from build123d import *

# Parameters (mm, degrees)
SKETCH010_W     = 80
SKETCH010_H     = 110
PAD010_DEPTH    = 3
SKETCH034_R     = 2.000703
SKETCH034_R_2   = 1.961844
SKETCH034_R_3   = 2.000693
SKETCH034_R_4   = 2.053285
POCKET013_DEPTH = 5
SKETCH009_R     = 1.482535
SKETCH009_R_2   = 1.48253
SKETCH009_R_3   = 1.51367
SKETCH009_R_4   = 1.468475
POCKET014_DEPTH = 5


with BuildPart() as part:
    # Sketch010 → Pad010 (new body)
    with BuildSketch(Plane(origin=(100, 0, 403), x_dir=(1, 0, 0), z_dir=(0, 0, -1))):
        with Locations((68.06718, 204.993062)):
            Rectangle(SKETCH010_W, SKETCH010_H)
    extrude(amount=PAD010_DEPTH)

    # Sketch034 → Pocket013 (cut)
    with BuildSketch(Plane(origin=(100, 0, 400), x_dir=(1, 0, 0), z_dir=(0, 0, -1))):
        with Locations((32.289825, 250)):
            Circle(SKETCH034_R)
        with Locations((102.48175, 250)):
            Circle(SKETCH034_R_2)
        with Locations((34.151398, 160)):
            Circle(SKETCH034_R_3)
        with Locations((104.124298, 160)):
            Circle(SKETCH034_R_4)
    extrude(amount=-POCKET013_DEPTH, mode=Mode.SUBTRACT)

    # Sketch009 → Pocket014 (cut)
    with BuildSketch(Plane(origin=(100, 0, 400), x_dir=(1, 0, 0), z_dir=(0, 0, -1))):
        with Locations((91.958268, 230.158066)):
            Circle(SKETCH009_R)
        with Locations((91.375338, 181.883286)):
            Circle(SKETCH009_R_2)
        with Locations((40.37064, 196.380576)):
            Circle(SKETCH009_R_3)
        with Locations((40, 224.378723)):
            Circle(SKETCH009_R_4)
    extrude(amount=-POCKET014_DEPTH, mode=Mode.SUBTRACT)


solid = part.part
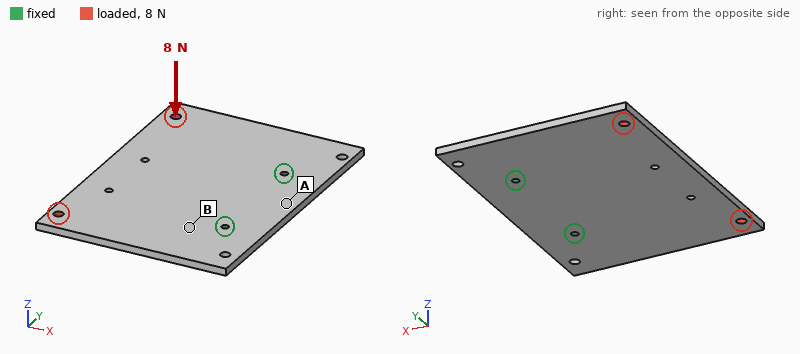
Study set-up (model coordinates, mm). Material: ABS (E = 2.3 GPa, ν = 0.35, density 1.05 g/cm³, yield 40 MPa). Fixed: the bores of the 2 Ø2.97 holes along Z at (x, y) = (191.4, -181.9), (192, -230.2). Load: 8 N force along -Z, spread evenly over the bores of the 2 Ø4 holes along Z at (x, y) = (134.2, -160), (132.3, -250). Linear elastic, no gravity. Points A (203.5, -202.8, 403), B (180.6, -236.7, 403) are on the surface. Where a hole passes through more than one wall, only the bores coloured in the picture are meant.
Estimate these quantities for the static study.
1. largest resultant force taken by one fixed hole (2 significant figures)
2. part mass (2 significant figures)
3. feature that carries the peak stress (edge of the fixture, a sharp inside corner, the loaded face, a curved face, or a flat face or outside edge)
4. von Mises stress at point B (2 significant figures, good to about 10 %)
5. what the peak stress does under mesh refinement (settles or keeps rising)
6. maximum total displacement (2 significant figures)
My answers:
4.2 N
27 g
edge of the fixture
2.3 MPa
keeps rising
1.5 mm
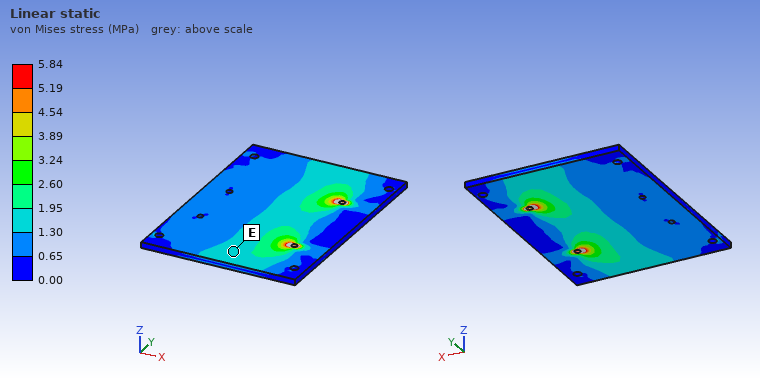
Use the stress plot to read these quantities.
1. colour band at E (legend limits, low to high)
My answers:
1.30 to 1.95 MPa
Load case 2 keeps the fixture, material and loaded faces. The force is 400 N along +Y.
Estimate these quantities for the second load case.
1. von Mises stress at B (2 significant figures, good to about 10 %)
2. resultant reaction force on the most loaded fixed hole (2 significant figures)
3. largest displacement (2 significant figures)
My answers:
3.4 MPa
520 N
0.47 mm
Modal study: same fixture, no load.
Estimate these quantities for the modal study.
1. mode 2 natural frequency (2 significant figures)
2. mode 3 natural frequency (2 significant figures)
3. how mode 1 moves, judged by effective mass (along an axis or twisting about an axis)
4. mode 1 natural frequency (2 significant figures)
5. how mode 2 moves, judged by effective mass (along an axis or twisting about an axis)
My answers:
240 Hz
480 Hz
along Z
150 Hz
twisting about X
